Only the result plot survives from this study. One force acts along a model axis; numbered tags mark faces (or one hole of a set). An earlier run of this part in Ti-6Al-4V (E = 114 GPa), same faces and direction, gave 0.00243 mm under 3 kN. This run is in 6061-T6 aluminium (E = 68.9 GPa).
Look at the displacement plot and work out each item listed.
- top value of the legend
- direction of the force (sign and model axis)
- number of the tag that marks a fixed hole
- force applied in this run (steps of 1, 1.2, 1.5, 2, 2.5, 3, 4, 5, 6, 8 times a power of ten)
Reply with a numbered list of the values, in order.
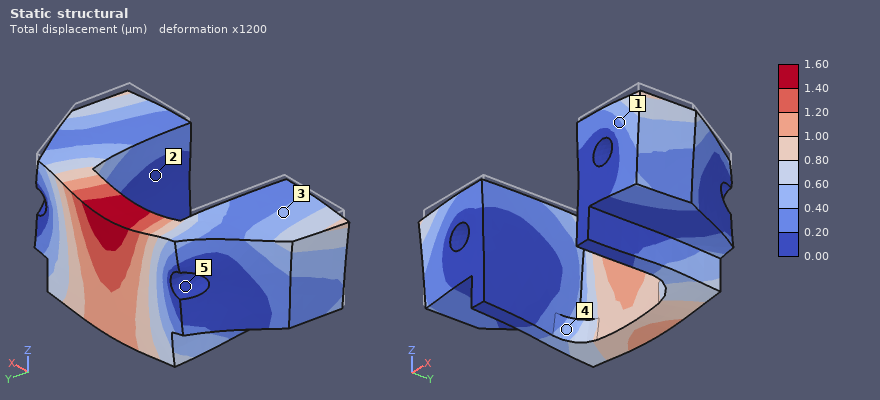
1. 1.60 µm
2. -Z
3. 5
4. 1.2 kN
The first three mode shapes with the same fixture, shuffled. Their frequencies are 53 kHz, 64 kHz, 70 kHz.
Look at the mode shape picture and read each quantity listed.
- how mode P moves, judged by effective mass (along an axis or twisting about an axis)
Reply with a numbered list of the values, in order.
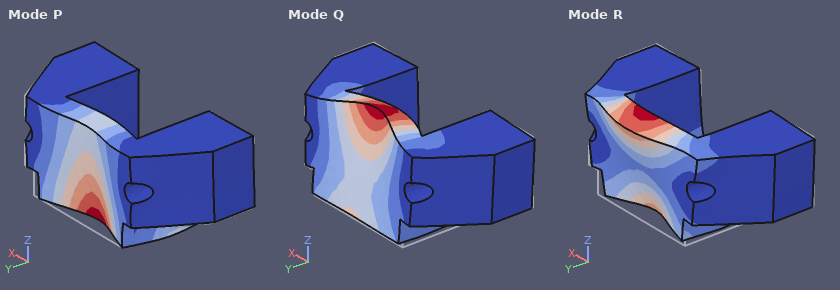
1. along Y
